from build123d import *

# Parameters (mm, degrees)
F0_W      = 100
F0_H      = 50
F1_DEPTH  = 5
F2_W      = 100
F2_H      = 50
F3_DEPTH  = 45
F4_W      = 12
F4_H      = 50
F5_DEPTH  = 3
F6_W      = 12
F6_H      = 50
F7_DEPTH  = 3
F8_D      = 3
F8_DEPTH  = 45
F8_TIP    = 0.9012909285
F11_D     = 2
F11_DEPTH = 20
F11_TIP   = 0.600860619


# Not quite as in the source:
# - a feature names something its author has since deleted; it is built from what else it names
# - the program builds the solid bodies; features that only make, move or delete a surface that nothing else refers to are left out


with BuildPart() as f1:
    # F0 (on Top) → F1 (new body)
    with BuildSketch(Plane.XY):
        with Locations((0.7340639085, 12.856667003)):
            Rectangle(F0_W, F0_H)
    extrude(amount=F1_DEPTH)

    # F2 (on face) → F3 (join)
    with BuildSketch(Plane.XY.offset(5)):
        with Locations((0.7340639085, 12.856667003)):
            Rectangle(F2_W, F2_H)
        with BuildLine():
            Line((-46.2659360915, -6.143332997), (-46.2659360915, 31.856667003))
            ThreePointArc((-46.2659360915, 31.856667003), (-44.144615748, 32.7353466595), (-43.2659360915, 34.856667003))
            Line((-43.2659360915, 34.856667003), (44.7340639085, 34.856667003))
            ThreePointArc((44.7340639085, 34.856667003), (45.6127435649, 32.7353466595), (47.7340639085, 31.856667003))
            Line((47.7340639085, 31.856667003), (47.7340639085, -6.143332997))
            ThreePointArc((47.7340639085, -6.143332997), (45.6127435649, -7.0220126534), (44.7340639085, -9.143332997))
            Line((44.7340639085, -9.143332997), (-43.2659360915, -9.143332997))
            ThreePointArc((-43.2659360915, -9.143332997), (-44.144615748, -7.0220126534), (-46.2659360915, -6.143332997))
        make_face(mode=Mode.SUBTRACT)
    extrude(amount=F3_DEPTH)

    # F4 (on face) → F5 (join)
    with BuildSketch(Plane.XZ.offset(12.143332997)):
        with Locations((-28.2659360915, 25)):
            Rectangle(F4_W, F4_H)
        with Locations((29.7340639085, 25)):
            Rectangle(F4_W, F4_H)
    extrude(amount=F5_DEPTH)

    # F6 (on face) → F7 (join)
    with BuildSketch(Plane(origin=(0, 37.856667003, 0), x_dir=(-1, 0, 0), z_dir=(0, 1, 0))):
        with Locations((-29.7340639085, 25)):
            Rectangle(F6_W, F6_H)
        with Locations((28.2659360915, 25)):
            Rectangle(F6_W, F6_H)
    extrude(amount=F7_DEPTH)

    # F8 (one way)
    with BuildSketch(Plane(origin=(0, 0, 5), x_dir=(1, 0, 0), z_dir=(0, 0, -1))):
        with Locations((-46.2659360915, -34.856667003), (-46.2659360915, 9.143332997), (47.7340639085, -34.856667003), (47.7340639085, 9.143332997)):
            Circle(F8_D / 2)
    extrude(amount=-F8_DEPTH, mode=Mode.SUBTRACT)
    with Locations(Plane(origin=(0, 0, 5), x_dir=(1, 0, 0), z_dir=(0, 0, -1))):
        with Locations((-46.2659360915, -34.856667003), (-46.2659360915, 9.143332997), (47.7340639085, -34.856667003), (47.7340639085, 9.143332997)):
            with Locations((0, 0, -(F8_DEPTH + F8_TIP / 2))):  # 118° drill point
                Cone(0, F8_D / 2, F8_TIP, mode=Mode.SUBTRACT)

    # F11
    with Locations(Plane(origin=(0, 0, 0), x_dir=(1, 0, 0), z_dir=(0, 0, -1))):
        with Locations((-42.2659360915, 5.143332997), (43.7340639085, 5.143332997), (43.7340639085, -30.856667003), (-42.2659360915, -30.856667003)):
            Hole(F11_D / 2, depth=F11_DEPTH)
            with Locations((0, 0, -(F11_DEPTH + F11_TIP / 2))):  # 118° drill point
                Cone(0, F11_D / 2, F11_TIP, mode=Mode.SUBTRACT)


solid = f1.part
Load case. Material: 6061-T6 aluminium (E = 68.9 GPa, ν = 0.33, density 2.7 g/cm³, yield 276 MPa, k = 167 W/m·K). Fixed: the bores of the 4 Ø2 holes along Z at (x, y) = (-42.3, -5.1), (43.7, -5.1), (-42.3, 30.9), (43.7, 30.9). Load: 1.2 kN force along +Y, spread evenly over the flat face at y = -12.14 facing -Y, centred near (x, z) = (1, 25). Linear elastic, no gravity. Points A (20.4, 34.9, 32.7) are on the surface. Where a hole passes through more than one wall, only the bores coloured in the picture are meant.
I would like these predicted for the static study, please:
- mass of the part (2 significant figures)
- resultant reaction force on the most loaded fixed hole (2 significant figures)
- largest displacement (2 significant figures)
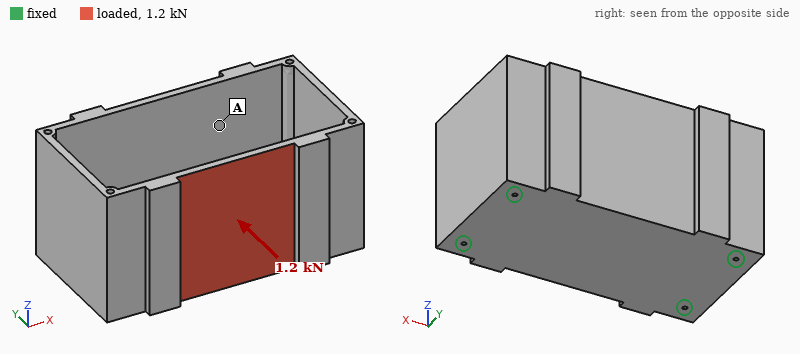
190 g
550 N
0.31 mm
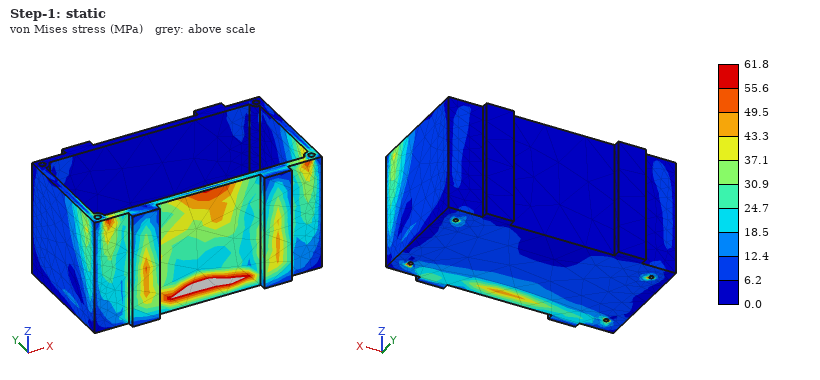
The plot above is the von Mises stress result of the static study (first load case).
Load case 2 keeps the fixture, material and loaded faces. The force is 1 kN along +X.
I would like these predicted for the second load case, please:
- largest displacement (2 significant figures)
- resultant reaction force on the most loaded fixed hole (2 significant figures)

7.0 µm
480 N
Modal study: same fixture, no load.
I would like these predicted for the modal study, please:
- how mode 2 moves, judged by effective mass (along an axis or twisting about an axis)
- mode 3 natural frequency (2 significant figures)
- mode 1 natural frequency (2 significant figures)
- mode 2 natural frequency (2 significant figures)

along Y
4100 Hz
2400 Hz
2600 Hz
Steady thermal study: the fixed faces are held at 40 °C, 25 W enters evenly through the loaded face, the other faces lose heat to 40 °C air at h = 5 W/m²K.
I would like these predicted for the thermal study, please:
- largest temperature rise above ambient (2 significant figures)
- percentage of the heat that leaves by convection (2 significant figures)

16 K
3.7 %
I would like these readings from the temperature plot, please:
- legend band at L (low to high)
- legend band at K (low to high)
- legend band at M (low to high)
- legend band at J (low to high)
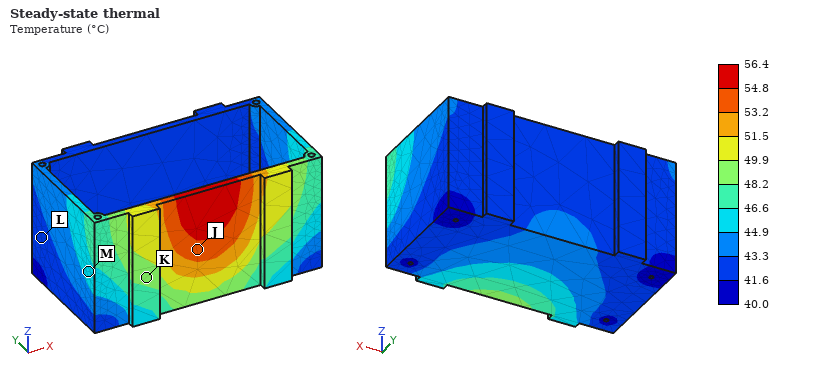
41.6 to 43.3 °C
48.2 to 49.9 °C
44.9 to 46.6 °C
53.2 to 54.8 °C
